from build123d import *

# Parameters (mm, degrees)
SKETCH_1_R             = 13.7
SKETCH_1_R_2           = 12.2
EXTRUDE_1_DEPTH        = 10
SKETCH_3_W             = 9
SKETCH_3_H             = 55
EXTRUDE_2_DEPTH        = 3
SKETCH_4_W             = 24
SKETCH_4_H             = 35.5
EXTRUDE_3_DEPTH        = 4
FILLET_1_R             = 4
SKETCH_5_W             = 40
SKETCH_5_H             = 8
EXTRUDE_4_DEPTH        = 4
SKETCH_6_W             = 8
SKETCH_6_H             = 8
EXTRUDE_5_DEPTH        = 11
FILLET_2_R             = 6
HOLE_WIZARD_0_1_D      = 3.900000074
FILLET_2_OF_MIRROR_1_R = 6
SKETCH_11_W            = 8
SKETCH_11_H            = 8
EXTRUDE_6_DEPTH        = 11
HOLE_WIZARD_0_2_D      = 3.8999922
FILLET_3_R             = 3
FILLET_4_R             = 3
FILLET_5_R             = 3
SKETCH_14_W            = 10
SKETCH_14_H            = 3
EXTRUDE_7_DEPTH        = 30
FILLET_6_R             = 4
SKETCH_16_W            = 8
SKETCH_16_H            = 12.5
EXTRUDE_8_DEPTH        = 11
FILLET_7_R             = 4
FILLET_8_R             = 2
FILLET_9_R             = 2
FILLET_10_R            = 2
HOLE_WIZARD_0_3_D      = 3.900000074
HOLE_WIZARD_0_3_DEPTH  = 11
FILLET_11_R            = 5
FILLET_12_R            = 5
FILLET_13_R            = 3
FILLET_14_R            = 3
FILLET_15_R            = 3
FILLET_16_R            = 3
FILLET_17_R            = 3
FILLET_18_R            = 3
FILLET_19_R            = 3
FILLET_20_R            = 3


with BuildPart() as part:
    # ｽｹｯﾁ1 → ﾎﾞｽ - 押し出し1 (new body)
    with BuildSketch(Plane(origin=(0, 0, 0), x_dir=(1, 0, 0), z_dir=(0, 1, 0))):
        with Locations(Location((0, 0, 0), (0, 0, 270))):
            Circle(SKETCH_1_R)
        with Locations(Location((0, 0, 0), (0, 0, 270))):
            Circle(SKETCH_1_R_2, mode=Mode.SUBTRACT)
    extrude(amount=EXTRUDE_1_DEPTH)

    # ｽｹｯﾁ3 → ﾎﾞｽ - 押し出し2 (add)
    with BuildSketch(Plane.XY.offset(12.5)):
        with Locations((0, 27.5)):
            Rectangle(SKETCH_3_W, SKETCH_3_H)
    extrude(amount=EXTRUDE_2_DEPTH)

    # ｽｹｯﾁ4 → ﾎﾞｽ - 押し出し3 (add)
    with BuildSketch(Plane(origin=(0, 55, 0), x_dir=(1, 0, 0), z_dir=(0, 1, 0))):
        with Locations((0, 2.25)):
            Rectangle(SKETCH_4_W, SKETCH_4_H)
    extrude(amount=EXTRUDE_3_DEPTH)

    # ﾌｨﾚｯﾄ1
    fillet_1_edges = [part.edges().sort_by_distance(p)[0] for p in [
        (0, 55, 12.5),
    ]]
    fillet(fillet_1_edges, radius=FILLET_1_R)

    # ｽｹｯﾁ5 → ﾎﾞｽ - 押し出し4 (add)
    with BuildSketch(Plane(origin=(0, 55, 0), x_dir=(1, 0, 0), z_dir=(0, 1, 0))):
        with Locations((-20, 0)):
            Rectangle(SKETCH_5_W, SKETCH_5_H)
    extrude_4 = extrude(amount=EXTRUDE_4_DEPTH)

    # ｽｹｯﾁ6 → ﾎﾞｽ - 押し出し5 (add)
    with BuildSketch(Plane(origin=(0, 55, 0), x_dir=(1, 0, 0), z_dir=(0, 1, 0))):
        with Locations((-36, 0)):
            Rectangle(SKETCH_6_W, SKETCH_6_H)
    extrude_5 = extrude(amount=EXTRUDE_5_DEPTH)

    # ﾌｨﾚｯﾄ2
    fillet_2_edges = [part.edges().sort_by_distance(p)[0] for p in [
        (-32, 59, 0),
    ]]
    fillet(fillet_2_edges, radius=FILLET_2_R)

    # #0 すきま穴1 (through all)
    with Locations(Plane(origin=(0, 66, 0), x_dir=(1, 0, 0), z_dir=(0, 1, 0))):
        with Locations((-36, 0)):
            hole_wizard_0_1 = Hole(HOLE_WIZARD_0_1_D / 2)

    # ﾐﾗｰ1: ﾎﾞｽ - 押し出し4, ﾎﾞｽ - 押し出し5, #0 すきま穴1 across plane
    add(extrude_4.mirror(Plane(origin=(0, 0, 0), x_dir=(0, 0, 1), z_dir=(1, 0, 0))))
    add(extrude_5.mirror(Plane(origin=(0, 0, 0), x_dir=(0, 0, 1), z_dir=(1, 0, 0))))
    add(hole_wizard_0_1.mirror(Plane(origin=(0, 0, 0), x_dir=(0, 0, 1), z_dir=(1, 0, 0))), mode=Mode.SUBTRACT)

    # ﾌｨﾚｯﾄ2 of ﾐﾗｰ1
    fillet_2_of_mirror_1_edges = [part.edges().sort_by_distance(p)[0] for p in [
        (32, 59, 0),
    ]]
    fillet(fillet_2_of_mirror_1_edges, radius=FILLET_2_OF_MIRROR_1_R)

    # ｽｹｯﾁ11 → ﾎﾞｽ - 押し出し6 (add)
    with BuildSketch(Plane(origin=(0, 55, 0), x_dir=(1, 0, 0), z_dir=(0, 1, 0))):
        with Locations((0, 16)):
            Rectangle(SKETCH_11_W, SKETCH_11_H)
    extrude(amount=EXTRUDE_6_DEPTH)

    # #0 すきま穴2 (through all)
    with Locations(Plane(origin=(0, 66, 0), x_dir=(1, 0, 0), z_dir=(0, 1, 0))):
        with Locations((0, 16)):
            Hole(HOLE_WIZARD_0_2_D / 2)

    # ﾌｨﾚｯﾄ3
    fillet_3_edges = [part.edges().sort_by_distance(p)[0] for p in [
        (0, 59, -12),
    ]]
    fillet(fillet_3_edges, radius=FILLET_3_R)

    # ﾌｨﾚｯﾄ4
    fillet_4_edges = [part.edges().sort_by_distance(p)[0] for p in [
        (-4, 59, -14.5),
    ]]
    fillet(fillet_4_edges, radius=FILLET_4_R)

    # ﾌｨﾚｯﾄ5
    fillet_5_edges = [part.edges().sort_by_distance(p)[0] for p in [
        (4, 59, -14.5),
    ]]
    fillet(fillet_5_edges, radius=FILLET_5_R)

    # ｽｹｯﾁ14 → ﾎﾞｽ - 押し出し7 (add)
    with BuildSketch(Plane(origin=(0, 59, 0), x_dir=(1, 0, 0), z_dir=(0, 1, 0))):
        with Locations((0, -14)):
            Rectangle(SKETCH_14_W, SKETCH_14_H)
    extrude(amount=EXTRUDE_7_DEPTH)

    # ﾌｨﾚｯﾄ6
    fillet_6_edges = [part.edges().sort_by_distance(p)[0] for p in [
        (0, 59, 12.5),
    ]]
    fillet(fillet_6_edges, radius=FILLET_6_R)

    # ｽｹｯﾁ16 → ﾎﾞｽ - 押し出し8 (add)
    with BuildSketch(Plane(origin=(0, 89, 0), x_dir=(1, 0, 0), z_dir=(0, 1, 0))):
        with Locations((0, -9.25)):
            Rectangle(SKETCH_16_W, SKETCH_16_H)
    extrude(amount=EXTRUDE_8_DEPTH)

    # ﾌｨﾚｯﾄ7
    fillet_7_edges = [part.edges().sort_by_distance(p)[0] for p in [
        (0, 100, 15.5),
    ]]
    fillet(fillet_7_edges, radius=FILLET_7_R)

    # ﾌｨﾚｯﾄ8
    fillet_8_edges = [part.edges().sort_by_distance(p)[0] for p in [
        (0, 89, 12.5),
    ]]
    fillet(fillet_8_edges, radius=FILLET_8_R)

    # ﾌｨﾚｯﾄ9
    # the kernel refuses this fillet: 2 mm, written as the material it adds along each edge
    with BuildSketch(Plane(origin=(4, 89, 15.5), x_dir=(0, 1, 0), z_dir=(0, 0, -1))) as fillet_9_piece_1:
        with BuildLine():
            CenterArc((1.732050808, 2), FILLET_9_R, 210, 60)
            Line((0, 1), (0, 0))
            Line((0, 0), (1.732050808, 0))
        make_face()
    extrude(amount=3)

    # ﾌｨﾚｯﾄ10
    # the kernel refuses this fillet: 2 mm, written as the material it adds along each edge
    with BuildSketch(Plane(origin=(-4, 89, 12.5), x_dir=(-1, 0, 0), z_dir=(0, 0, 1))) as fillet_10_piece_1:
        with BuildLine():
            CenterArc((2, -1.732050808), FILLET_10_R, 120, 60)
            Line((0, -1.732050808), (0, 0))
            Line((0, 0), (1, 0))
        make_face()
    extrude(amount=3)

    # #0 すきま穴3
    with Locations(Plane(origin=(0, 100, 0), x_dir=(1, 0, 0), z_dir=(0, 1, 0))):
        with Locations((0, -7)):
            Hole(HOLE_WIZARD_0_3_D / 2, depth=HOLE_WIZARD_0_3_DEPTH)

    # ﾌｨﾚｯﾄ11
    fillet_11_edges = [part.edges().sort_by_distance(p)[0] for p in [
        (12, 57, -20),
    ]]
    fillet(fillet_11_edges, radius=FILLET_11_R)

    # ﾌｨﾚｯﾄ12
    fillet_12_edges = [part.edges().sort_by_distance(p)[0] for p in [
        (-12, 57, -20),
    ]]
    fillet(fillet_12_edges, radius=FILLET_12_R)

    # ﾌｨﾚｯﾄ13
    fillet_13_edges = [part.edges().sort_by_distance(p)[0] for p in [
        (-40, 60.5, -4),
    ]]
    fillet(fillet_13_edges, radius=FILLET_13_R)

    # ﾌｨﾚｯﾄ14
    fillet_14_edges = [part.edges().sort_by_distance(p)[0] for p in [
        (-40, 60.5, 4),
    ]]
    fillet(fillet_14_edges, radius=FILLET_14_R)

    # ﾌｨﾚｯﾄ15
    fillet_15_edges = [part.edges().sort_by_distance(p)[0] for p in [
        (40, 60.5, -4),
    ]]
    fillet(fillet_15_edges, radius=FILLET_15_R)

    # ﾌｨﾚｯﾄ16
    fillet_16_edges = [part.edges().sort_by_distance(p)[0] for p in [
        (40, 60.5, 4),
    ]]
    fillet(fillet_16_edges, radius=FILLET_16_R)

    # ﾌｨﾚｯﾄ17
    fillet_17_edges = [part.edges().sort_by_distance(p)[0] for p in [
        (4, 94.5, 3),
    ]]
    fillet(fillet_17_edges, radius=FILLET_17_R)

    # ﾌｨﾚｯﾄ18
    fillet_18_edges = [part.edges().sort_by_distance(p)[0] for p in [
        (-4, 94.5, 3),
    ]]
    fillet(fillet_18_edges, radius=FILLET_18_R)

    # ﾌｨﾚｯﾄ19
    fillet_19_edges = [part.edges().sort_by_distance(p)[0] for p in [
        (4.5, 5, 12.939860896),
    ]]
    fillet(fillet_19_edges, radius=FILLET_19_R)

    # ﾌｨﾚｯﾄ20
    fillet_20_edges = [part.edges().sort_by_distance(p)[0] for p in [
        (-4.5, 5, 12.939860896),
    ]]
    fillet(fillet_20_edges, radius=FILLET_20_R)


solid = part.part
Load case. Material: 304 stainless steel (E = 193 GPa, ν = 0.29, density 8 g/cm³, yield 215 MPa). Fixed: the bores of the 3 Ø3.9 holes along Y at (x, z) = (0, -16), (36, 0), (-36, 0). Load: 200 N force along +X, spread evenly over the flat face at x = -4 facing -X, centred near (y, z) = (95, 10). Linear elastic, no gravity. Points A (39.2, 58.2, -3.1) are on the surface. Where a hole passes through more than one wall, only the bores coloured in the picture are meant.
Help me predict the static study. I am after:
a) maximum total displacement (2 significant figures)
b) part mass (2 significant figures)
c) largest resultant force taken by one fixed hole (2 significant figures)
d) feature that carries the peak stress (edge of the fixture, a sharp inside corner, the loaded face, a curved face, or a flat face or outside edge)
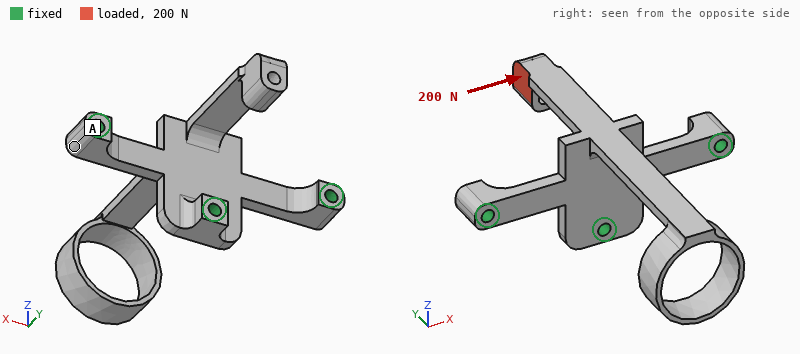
0.26 mm
86 g
160 N
a curved face
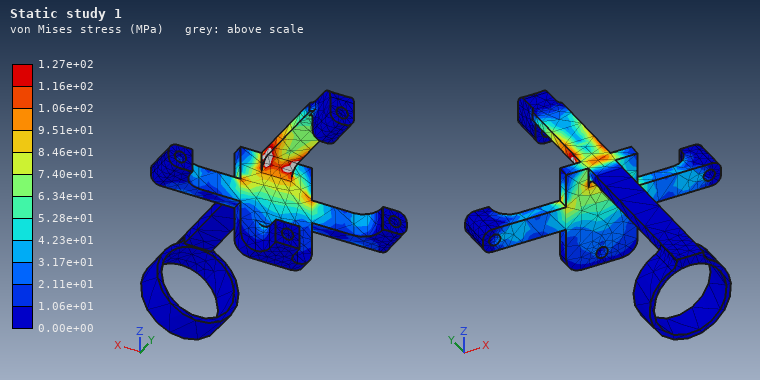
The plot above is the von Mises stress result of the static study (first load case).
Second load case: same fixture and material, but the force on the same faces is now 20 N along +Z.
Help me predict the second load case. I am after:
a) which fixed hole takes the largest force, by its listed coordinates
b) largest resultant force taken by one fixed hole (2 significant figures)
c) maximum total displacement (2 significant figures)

(0, -16)
25 N
0.11 mm
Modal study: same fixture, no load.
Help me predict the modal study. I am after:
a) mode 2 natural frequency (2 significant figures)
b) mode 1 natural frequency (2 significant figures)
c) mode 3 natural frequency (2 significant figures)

630 Hz
370 Hz
830 Hz
